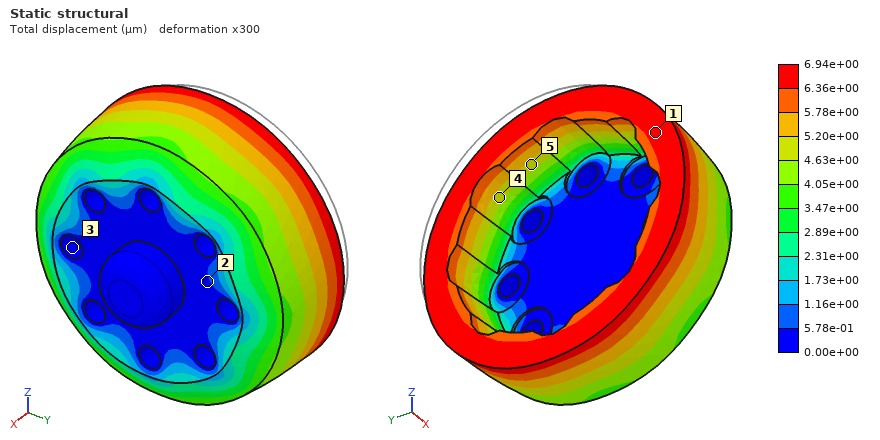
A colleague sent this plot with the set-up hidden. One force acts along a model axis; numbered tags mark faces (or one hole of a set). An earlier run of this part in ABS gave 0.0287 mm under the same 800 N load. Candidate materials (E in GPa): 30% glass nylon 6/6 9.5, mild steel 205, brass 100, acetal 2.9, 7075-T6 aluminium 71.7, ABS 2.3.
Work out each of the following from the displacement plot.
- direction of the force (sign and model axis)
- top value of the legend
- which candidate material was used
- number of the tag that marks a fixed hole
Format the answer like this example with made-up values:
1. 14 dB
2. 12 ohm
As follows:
1. +X
2. 6.94e+00 µm
3. 30% glass nylon 6/6
4. 3
